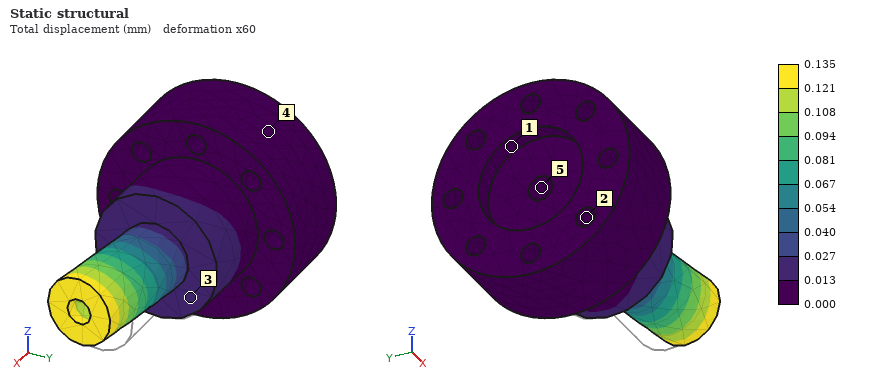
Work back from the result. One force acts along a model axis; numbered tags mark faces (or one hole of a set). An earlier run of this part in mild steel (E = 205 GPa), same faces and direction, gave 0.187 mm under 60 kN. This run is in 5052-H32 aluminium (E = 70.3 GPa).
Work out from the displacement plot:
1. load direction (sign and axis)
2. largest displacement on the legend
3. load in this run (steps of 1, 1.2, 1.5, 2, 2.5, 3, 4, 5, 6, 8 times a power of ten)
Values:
-Y
0.135 mm
15 kN
